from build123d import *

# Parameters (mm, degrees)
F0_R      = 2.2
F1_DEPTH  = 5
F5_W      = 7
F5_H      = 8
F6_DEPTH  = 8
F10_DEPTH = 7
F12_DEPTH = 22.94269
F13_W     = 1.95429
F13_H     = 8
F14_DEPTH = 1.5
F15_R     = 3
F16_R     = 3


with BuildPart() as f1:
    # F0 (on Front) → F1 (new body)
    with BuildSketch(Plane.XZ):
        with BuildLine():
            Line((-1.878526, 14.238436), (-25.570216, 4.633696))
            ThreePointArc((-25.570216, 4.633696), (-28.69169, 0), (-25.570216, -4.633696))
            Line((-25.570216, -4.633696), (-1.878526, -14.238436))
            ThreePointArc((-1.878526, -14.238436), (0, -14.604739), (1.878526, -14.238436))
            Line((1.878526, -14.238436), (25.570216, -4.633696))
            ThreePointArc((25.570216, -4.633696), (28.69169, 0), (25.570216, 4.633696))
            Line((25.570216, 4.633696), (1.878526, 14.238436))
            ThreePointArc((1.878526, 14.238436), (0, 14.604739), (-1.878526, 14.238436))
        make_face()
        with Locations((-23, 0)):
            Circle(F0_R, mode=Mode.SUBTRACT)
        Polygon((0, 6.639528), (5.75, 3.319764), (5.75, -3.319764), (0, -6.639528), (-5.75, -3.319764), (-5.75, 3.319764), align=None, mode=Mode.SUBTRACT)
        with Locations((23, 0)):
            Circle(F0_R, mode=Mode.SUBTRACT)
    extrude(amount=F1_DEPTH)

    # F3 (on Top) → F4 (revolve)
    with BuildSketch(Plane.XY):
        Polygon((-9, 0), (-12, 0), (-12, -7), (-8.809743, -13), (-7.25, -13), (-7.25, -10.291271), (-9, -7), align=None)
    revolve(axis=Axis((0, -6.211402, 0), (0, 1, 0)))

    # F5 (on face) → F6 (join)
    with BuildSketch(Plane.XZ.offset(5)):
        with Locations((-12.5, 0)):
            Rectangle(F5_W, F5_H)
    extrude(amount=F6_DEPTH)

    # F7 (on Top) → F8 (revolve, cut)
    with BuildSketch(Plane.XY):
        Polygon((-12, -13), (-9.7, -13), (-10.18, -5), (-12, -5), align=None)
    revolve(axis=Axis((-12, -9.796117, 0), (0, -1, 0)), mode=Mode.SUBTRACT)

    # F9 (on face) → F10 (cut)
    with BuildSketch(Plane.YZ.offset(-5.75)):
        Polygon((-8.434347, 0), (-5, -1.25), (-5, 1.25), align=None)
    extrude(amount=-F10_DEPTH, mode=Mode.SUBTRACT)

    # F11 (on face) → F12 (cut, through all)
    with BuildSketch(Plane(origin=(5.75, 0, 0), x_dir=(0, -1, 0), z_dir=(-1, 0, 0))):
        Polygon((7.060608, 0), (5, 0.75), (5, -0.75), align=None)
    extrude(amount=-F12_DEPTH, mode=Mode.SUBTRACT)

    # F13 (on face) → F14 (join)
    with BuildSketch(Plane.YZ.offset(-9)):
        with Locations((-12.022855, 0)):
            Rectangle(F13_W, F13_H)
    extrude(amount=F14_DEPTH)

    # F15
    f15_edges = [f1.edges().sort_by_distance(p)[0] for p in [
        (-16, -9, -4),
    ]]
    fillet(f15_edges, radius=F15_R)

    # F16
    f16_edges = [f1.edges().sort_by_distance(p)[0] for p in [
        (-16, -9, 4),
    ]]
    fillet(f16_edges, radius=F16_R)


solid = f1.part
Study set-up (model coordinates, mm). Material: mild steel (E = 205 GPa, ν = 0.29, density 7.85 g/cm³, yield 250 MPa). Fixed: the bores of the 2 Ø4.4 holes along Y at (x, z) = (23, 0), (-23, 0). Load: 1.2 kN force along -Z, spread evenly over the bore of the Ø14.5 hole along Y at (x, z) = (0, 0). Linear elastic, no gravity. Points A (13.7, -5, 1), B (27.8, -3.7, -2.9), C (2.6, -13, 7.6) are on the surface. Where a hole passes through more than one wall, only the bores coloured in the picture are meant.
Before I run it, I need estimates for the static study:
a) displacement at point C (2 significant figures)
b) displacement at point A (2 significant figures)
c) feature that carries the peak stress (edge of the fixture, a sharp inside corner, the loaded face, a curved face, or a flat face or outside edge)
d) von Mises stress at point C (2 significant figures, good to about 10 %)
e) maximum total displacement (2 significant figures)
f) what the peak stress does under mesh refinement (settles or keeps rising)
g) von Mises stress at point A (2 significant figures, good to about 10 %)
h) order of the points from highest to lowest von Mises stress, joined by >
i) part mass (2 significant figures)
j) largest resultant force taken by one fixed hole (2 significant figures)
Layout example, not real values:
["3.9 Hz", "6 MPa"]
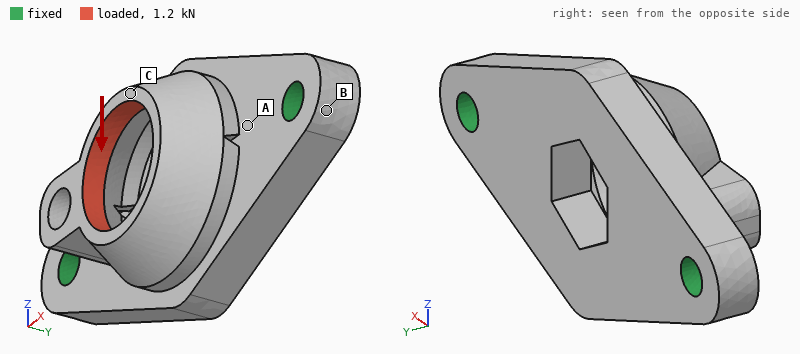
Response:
["21 µm", "4.1 µm", "edge of the fixture", "31 MPa", "22 µm", "keeps rising", "66 MPa", "A > C > B", "47 g", "610 N"]
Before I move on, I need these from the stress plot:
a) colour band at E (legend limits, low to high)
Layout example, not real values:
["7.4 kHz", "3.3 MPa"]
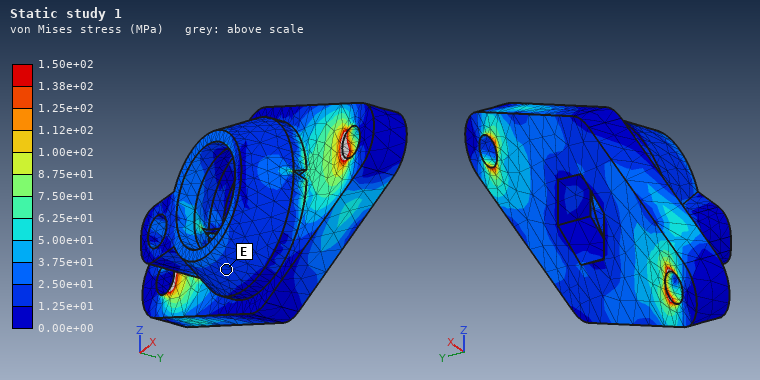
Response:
["1.25e+01 to 2.50e+01 MPa"]
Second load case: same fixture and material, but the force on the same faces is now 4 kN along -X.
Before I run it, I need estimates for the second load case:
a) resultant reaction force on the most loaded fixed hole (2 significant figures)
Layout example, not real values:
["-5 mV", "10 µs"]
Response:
["2.3 kN"]
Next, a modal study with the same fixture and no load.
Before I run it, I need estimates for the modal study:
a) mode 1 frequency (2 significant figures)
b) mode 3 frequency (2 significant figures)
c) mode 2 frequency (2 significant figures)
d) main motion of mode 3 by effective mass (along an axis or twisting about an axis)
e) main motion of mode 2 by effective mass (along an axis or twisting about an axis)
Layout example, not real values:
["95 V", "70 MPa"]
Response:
["9100 Hz", "21 kHz", "11 kHz", "along Z", "along Y"]
